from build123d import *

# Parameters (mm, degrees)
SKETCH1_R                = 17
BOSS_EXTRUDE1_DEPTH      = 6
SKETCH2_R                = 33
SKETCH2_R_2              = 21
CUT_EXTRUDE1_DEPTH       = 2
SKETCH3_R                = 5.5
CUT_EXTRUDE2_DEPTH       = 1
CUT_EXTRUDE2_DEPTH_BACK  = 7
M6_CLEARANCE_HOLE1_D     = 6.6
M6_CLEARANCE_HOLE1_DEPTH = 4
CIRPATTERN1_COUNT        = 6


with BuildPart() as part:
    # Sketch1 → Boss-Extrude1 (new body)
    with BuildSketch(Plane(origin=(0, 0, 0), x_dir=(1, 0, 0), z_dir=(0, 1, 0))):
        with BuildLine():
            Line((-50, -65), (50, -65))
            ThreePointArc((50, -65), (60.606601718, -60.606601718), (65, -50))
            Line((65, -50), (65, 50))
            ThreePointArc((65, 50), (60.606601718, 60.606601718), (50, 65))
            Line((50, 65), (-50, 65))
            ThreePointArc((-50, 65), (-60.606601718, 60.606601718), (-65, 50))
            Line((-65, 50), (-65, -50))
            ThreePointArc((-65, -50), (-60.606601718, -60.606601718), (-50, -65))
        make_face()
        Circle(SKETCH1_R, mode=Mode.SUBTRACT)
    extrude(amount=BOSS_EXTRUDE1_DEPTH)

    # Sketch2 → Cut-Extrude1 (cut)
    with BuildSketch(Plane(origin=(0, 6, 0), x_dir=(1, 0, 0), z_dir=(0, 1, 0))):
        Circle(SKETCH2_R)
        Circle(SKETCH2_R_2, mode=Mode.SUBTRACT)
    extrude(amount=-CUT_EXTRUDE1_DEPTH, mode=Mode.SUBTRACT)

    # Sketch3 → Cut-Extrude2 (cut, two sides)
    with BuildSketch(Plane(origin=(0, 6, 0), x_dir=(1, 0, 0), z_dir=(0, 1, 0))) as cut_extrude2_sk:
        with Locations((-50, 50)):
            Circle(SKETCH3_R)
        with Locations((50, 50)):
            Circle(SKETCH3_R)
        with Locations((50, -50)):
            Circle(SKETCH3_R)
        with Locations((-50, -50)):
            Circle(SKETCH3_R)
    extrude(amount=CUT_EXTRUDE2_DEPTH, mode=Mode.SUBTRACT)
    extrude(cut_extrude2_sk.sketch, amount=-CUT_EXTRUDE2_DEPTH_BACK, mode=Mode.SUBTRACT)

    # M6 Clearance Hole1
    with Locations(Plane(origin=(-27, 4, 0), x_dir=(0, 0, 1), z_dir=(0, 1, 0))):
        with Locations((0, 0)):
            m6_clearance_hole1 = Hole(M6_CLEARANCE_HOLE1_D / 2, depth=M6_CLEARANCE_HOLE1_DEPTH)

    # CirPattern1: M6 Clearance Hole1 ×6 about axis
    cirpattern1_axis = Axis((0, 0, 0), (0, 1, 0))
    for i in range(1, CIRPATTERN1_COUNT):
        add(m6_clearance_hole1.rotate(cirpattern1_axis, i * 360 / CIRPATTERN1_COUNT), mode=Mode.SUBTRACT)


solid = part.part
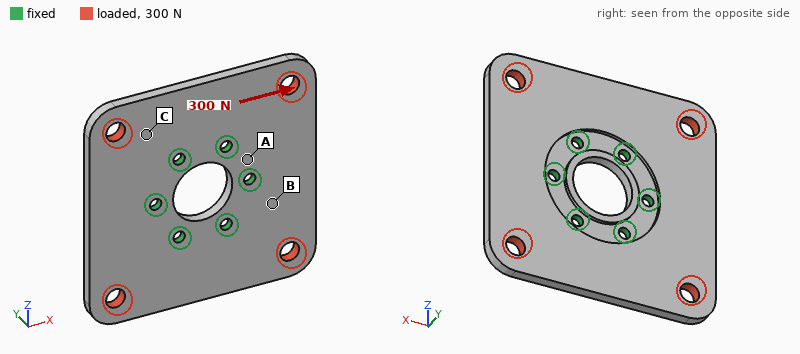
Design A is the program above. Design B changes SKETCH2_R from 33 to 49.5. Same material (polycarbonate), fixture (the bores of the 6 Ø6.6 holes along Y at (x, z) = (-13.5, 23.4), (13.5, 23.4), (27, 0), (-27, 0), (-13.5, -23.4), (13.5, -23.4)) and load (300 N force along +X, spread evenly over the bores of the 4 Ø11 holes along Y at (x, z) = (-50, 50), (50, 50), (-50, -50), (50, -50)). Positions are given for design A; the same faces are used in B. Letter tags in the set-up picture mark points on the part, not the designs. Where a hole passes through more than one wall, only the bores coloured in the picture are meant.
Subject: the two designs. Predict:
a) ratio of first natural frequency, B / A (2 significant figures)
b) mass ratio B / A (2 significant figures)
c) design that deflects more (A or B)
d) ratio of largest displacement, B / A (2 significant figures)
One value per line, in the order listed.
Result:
0.82
0.90
B
2.4
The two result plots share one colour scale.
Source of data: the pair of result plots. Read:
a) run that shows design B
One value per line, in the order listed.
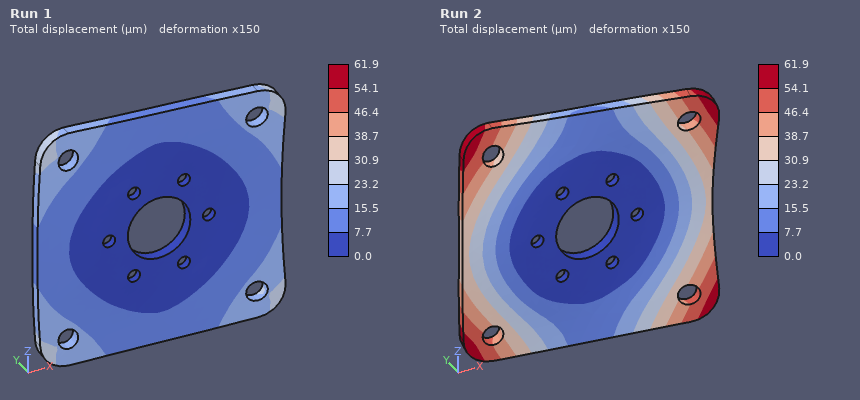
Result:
Run 2
